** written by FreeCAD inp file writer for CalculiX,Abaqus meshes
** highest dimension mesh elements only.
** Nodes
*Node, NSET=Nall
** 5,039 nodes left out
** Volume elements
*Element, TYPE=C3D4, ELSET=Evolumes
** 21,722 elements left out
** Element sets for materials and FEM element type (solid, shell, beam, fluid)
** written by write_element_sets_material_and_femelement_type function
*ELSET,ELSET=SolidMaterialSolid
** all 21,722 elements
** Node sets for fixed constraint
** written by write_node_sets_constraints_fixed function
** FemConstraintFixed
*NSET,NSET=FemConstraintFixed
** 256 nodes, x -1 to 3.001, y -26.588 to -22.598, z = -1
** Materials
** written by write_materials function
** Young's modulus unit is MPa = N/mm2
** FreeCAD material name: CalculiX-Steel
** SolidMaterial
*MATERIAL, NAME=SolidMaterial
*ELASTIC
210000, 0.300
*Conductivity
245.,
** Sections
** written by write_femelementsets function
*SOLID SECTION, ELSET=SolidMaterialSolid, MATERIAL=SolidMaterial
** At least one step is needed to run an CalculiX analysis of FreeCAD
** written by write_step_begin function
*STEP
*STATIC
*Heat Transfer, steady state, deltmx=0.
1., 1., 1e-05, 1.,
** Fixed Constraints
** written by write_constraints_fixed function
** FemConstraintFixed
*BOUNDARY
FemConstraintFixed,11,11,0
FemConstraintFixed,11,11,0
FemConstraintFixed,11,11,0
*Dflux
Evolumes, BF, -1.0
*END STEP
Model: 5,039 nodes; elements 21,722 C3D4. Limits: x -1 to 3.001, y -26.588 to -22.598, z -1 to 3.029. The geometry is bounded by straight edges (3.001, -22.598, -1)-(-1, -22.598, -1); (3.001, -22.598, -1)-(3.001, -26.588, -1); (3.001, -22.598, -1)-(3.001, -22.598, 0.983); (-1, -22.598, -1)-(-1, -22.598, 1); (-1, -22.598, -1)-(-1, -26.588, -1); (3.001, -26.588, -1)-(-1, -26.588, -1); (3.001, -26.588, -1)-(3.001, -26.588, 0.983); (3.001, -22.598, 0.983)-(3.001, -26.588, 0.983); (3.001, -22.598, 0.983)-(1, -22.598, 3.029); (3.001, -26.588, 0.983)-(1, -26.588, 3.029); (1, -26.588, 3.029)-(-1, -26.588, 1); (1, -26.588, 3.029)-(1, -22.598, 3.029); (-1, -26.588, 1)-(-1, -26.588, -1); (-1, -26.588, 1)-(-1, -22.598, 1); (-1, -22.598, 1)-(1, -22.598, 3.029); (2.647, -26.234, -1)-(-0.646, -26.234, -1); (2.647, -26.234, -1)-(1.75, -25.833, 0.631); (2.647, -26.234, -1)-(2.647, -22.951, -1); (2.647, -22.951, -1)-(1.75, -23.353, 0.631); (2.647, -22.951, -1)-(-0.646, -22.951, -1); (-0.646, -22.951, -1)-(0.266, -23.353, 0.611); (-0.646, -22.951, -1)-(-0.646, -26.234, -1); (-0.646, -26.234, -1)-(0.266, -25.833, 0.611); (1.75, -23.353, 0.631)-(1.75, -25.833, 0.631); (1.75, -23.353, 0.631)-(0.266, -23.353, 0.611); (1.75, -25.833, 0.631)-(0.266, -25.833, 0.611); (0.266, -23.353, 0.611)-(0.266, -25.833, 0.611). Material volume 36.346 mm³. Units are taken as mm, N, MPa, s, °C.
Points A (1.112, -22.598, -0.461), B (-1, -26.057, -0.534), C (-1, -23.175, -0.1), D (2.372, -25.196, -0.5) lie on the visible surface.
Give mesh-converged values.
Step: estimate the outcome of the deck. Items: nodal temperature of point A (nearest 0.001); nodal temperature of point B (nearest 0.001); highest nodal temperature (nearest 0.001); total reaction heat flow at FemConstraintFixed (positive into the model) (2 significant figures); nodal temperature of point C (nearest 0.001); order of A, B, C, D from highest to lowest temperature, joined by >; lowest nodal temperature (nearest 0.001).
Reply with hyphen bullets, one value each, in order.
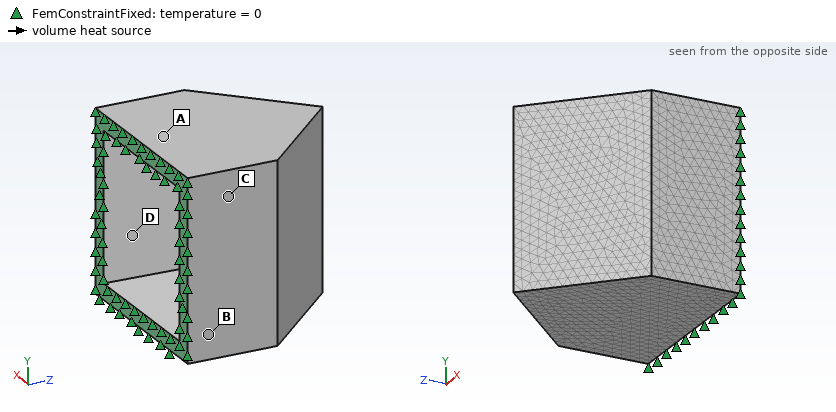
- -0.012 °C
- -0.010 °C
- 0.000 °C
- 36 mW
- -0.017 °C
- B > A > D > C
- -0.034 °C
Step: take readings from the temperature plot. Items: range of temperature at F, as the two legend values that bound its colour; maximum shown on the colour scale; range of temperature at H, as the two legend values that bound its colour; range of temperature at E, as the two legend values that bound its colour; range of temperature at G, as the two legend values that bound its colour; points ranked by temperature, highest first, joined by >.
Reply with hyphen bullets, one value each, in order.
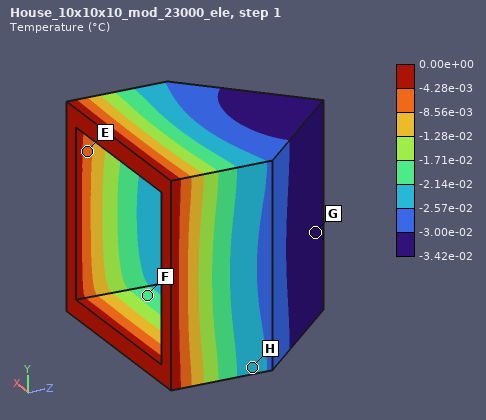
- -2.14e-02 to -1.71e-02 °C
- 0.00e+00 °C
- -2.57e-02 to -2.14e-02 °C
- -8.56e-03 to -4.28e-03 °C
- -3.42e-02 to -3.00e-02 °C
- E > F > H > G
